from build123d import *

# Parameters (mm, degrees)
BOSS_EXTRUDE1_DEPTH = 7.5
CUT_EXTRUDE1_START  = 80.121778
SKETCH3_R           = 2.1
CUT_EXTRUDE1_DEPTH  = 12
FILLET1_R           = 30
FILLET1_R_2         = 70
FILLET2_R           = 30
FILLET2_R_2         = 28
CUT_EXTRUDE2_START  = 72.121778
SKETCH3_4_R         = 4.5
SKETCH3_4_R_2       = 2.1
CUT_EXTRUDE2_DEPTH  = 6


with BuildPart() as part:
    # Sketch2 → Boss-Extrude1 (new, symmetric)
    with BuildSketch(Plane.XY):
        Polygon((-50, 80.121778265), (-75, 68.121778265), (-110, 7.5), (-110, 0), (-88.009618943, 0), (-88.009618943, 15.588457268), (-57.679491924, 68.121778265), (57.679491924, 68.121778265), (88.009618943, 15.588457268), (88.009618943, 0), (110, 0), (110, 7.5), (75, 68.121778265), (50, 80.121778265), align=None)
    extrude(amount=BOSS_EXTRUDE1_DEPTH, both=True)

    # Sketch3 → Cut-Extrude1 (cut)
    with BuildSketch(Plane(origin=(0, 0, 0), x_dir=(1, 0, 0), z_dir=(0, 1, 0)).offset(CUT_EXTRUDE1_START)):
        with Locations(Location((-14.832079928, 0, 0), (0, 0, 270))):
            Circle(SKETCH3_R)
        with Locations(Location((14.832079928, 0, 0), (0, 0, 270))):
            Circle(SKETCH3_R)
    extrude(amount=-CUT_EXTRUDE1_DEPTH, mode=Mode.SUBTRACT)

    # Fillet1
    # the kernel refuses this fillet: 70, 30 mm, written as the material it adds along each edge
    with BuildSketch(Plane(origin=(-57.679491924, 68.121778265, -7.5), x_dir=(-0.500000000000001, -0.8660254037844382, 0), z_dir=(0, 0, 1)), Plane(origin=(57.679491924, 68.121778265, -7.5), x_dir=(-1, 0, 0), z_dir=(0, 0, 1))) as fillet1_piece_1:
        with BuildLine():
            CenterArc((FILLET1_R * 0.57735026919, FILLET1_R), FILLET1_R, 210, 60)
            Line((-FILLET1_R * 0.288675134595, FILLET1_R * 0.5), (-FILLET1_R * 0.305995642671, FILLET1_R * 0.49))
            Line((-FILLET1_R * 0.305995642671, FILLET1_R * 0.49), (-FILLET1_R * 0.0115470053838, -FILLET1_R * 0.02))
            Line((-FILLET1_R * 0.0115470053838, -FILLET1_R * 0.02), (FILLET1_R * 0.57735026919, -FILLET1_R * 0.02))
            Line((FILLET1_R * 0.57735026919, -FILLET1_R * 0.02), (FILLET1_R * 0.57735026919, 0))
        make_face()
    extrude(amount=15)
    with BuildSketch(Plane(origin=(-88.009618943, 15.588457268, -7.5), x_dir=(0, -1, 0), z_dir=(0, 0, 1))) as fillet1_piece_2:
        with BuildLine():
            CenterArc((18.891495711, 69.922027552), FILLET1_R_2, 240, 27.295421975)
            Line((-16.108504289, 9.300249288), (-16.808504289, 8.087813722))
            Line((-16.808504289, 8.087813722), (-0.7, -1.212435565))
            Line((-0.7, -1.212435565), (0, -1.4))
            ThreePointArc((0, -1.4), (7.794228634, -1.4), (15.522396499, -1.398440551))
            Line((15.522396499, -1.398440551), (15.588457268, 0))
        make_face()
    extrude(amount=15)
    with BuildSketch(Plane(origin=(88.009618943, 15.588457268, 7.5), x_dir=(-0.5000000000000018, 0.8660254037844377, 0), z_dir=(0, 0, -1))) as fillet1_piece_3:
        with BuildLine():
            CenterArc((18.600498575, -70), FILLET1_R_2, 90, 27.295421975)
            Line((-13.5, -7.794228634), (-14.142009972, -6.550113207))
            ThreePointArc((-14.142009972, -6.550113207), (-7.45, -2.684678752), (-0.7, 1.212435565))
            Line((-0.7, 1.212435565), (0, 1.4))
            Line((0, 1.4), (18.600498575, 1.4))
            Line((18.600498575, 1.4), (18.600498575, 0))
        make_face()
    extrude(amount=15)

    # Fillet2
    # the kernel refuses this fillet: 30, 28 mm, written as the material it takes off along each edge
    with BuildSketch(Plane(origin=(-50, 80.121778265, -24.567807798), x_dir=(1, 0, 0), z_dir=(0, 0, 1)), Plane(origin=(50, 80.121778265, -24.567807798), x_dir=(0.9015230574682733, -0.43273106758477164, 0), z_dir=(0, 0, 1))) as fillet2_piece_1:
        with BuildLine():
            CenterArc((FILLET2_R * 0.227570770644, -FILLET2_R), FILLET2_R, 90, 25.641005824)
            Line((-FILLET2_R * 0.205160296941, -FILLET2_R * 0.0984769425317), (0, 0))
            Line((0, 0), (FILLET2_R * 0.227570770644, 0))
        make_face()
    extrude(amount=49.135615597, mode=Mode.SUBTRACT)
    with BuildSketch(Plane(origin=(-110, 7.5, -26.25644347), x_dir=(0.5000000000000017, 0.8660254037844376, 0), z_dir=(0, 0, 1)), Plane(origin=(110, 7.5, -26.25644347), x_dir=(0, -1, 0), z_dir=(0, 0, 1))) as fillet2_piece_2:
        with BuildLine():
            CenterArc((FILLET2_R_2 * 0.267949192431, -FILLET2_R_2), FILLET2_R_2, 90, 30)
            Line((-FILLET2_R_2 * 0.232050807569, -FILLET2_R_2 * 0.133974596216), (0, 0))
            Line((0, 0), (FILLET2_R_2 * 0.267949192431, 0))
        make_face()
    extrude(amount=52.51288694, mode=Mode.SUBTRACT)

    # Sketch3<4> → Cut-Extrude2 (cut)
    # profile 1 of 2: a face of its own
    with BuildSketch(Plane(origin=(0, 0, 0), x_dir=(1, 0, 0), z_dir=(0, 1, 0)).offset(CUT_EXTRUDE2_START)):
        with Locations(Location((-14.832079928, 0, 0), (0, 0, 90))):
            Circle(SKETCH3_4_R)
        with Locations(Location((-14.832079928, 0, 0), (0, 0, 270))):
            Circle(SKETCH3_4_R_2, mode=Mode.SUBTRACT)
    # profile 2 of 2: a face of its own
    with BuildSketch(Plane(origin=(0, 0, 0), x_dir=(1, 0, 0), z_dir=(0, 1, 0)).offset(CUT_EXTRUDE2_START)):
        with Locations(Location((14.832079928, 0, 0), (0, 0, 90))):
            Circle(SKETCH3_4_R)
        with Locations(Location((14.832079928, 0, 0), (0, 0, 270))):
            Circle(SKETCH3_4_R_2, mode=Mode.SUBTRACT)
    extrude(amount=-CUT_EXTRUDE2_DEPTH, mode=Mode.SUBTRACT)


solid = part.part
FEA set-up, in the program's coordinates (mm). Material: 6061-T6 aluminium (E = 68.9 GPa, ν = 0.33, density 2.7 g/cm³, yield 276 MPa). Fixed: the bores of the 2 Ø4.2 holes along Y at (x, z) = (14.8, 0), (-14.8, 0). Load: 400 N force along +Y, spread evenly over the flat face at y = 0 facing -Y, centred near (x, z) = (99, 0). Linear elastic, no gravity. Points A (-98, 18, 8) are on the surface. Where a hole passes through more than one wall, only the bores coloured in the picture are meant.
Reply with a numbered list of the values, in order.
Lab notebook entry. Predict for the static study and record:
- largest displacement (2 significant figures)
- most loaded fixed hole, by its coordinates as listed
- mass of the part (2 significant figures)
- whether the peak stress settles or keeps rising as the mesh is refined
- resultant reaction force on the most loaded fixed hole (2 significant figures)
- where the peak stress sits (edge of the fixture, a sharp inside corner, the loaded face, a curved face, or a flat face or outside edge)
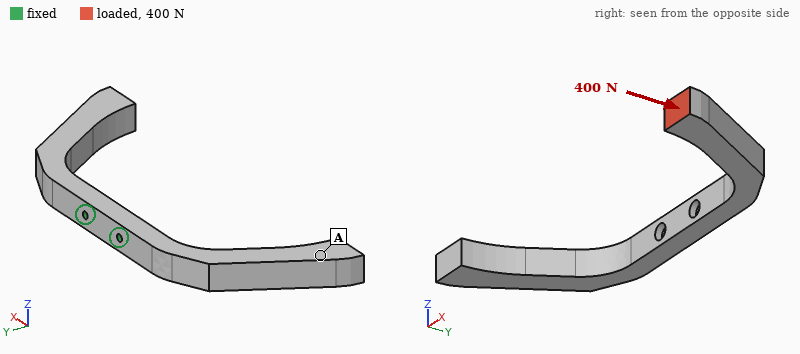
1. 1.1 mm
2. (14.8, 0)
3. 160 g
4. keeps rising
5. 1.1 kN
6. edge of the fixture
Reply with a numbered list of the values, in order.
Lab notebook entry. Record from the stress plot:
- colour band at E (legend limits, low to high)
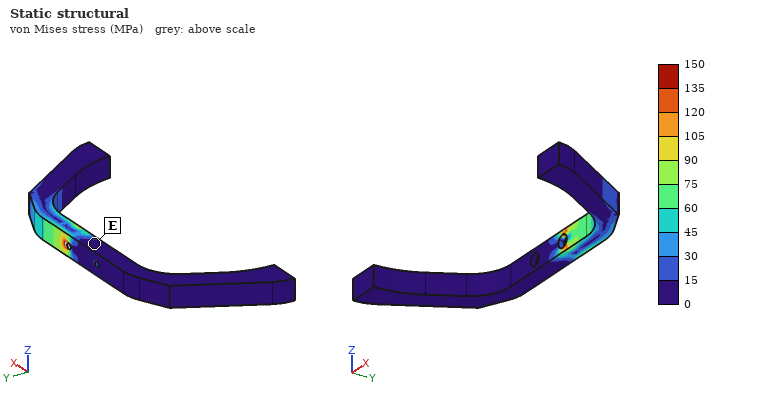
1. 0 to 15 MPa
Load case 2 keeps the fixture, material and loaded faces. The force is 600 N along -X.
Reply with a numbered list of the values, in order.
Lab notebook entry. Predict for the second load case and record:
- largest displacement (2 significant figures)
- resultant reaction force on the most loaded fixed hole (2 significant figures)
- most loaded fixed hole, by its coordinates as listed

1. 2.0 mm
2. 1.1 kN
3. (-14.8, 0)
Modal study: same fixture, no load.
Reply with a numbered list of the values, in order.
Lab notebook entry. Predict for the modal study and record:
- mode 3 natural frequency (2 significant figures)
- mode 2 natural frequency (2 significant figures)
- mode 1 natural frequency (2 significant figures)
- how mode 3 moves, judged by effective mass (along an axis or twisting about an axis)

1. 540 Hz
2. 510 Hz
3. 500 Hz
4. along Z
